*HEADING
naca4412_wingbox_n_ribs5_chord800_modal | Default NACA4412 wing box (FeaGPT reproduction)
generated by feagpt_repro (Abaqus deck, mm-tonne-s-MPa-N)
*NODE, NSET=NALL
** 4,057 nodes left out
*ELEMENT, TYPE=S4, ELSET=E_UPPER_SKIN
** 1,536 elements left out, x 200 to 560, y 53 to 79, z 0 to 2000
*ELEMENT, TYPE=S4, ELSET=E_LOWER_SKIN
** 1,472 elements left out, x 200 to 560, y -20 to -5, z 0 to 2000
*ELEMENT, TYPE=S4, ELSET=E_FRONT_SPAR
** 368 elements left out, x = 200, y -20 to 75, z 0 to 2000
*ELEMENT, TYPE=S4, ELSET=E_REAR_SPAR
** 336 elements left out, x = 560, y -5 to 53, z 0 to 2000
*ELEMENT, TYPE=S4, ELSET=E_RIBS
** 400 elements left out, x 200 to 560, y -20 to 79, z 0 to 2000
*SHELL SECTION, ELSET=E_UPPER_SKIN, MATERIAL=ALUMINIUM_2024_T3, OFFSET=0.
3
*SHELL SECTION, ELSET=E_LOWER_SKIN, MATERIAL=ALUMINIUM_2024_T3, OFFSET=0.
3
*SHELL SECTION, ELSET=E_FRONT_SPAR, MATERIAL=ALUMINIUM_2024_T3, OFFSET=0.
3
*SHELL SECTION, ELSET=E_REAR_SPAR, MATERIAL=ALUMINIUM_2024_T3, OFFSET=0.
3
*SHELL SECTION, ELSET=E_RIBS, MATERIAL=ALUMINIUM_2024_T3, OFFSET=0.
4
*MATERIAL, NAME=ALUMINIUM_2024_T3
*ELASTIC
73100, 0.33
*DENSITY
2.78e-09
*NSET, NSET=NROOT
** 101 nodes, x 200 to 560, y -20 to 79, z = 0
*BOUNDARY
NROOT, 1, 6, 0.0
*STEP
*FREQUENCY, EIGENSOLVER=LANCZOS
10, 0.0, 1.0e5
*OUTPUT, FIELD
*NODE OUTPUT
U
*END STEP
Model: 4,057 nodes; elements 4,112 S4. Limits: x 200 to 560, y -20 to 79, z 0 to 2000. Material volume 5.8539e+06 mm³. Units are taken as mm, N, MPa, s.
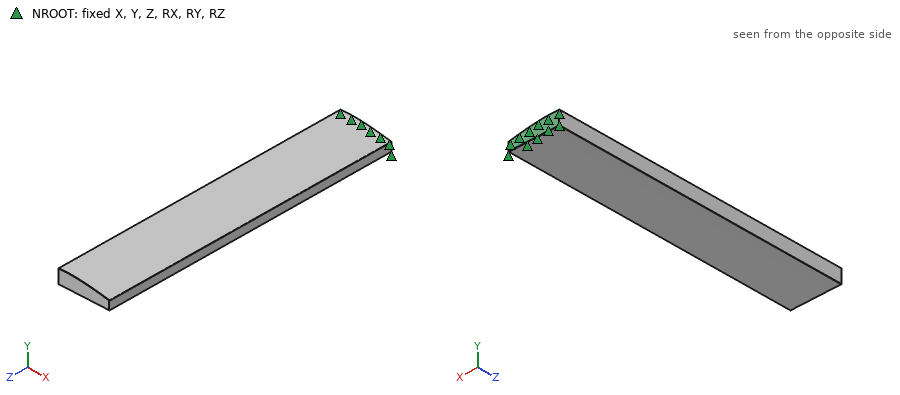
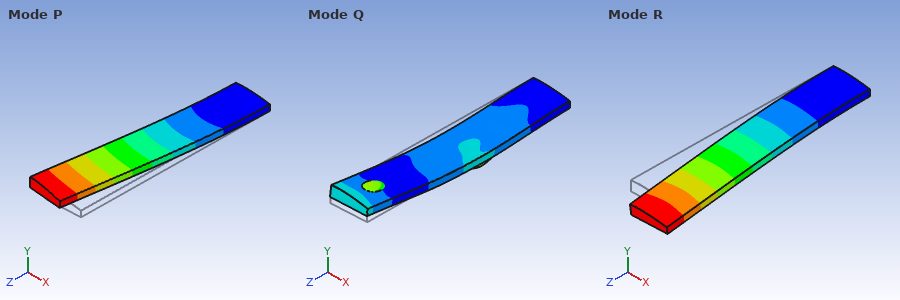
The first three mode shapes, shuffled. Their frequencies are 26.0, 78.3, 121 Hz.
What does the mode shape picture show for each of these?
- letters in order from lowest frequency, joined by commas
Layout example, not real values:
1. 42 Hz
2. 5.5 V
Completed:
1. R, P, Q
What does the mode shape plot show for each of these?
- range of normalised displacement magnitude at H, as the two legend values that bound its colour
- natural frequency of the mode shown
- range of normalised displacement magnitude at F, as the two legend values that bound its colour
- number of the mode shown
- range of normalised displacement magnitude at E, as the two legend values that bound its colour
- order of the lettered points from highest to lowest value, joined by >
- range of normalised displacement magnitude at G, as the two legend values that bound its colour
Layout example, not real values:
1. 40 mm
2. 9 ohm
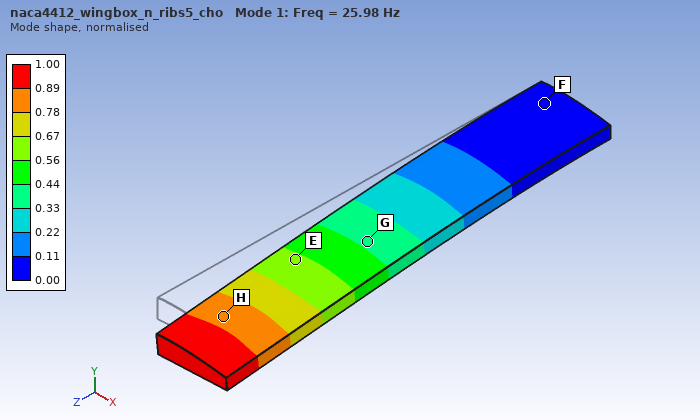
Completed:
1. 0.78 to 0.89
2. 25.98 Hz
3. 0.00 to 0.11
4. 1
5. 0.56 to 0.67
6. H > E > G > F
7. 0.33 to 0.44
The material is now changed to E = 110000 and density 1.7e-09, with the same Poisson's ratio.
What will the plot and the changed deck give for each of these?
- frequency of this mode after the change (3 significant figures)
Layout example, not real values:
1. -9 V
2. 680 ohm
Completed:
1. 40.8 Hz
